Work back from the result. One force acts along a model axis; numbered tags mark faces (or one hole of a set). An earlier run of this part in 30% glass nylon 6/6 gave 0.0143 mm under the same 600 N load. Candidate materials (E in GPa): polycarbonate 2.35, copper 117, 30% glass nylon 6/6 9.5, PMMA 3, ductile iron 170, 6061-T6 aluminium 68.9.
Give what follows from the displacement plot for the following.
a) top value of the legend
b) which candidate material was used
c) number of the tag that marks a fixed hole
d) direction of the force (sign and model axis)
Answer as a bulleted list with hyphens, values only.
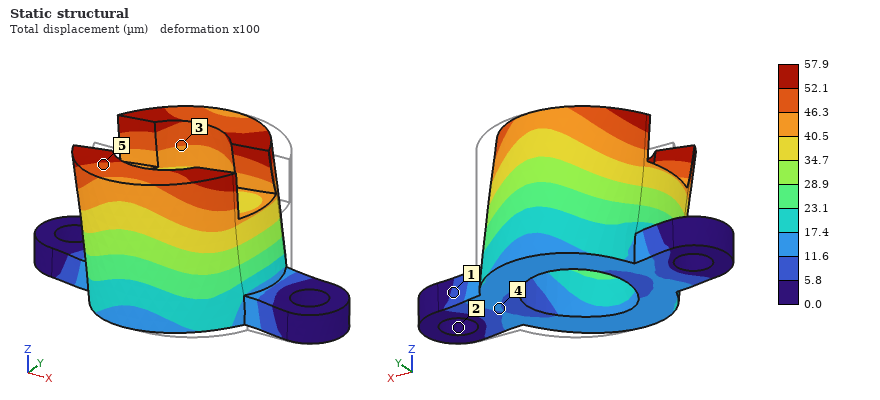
- 57.9 µm
- polycarbonate
- 2
- -X
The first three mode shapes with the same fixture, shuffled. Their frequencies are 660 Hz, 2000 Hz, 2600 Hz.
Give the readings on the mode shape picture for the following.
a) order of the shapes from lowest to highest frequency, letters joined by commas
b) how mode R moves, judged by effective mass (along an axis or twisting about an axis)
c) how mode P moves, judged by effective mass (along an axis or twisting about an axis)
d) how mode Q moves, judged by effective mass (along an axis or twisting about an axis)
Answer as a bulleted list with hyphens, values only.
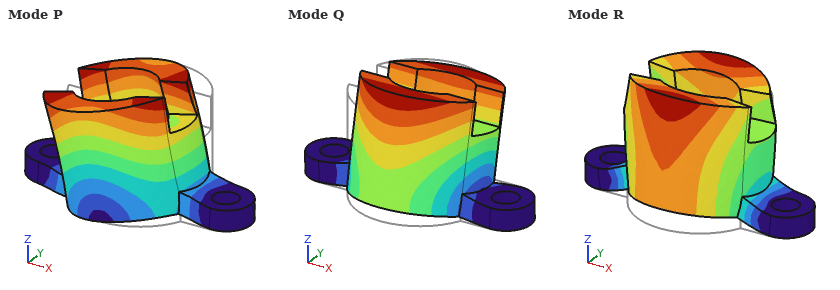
- Q, R, P
- along Z
- along X
- along Y
